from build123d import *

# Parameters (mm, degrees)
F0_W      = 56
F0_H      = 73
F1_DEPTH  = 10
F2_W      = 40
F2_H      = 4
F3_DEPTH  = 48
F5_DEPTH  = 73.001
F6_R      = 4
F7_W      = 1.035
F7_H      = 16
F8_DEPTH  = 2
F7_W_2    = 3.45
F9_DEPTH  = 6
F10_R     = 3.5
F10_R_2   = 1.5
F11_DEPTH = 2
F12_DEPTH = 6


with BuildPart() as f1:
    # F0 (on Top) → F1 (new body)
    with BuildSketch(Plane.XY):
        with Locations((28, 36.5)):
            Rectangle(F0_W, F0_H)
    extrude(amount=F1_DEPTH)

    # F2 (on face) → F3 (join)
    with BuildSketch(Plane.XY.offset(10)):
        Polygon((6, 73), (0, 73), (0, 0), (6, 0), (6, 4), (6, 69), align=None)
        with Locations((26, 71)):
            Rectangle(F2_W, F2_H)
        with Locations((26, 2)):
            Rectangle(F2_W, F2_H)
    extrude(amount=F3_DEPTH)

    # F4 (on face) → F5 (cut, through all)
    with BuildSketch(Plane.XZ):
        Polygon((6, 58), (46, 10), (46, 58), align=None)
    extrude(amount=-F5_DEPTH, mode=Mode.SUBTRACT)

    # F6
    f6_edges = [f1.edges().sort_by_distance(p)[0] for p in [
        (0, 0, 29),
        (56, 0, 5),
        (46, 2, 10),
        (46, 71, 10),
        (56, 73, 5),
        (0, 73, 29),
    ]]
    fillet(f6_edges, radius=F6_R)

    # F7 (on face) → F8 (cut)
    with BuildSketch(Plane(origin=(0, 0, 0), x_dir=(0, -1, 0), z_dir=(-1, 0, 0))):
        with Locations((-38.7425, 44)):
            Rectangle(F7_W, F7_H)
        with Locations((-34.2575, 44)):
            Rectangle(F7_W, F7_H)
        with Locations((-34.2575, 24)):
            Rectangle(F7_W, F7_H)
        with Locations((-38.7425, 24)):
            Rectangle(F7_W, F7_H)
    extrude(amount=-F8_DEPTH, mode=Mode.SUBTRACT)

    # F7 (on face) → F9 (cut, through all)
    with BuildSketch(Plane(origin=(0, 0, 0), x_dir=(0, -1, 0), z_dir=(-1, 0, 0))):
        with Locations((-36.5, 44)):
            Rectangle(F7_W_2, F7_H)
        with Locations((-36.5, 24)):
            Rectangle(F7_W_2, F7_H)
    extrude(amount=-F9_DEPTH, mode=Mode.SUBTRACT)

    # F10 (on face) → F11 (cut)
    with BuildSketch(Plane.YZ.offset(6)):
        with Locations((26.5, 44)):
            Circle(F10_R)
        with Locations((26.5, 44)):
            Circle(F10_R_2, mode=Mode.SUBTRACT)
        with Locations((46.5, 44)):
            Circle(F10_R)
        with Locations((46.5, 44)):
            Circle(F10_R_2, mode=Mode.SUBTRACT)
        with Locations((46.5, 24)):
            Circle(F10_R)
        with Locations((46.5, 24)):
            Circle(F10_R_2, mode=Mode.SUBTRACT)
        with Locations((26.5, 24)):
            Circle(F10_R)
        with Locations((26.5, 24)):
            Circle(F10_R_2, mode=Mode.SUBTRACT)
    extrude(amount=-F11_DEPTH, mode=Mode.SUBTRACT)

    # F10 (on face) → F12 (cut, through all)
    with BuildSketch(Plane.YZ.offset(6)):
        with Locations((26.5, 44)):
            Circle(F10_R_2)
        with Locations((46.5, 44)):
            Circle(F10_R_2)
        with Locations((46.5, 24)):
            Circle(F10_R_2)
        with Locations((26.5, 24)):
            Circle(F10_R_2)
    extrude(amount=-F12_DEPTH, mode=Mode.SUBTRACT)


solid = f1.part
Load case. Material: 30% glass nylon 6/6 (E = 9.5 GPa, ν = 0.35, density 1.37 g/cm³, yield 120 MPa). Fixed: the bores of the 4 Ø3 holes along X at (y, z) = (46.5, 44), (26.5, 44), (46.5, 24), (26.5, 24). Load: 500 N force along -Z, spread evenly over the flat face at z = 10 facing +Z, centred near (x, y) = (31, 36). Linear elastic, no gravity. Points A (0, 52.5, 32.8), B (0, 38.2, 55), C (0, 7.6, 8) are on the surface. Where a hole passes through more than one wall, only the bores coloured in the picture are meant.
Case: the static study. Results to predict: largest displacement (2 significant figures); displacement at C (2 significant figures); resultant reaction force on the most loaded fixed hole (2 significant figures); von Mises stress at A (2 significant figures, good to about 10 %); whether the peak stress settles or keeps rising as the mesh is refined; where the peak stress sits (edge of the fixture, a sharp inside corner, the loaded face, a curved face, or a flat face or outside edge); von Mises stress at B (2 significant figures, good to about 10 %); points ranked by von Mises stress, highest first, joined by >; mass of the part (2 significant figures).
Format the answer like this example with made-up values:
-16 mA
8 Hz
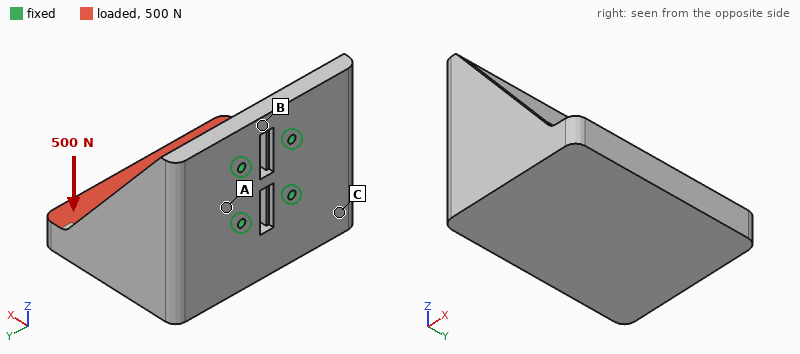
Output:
0.58 mm
0.13 mm
370 N
9.5 MPa
keeps rising
edge of the fixture
15 MPa
B > A > C
93 g
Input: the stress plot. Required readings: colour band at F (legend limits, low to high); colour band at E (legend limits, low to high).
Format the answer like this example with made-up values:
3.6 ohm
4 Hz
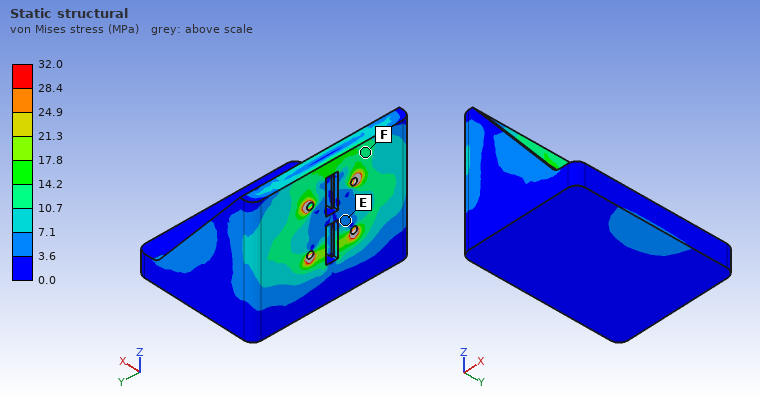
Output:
10.7 to 14.2 MPa
3.6 to 7.1 MPa
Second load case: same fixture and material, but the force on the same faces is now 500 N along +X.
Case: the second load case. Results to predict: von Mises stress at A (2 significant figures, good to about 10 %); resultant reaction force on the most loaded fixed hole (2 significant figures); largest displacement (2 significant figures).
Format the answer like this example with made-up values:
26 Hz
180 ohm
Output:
4.7 MPa
380 N
0.22 mm
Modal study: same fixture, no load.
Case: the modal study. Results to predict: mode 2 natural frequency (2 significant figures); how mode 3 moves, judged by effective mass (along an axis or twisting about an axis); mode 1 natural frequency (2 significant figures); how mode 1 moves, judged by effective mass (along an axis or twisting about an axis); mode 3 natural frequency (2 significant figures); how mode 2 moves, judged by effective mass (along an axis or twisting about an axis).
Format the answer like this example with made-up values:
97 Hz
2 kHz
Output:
780 Hz
along X
720 Hz
along Z
2000 Hz
along Y
